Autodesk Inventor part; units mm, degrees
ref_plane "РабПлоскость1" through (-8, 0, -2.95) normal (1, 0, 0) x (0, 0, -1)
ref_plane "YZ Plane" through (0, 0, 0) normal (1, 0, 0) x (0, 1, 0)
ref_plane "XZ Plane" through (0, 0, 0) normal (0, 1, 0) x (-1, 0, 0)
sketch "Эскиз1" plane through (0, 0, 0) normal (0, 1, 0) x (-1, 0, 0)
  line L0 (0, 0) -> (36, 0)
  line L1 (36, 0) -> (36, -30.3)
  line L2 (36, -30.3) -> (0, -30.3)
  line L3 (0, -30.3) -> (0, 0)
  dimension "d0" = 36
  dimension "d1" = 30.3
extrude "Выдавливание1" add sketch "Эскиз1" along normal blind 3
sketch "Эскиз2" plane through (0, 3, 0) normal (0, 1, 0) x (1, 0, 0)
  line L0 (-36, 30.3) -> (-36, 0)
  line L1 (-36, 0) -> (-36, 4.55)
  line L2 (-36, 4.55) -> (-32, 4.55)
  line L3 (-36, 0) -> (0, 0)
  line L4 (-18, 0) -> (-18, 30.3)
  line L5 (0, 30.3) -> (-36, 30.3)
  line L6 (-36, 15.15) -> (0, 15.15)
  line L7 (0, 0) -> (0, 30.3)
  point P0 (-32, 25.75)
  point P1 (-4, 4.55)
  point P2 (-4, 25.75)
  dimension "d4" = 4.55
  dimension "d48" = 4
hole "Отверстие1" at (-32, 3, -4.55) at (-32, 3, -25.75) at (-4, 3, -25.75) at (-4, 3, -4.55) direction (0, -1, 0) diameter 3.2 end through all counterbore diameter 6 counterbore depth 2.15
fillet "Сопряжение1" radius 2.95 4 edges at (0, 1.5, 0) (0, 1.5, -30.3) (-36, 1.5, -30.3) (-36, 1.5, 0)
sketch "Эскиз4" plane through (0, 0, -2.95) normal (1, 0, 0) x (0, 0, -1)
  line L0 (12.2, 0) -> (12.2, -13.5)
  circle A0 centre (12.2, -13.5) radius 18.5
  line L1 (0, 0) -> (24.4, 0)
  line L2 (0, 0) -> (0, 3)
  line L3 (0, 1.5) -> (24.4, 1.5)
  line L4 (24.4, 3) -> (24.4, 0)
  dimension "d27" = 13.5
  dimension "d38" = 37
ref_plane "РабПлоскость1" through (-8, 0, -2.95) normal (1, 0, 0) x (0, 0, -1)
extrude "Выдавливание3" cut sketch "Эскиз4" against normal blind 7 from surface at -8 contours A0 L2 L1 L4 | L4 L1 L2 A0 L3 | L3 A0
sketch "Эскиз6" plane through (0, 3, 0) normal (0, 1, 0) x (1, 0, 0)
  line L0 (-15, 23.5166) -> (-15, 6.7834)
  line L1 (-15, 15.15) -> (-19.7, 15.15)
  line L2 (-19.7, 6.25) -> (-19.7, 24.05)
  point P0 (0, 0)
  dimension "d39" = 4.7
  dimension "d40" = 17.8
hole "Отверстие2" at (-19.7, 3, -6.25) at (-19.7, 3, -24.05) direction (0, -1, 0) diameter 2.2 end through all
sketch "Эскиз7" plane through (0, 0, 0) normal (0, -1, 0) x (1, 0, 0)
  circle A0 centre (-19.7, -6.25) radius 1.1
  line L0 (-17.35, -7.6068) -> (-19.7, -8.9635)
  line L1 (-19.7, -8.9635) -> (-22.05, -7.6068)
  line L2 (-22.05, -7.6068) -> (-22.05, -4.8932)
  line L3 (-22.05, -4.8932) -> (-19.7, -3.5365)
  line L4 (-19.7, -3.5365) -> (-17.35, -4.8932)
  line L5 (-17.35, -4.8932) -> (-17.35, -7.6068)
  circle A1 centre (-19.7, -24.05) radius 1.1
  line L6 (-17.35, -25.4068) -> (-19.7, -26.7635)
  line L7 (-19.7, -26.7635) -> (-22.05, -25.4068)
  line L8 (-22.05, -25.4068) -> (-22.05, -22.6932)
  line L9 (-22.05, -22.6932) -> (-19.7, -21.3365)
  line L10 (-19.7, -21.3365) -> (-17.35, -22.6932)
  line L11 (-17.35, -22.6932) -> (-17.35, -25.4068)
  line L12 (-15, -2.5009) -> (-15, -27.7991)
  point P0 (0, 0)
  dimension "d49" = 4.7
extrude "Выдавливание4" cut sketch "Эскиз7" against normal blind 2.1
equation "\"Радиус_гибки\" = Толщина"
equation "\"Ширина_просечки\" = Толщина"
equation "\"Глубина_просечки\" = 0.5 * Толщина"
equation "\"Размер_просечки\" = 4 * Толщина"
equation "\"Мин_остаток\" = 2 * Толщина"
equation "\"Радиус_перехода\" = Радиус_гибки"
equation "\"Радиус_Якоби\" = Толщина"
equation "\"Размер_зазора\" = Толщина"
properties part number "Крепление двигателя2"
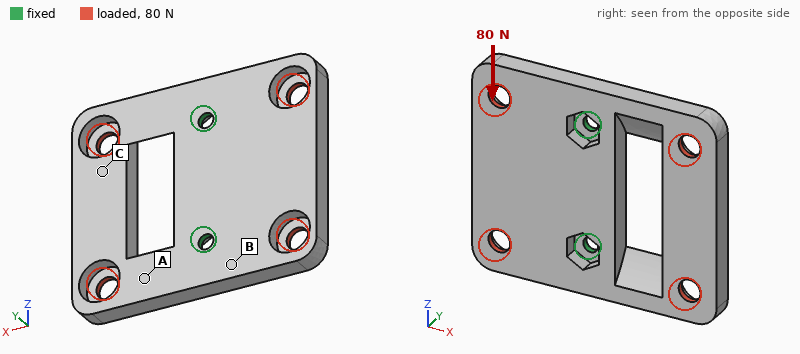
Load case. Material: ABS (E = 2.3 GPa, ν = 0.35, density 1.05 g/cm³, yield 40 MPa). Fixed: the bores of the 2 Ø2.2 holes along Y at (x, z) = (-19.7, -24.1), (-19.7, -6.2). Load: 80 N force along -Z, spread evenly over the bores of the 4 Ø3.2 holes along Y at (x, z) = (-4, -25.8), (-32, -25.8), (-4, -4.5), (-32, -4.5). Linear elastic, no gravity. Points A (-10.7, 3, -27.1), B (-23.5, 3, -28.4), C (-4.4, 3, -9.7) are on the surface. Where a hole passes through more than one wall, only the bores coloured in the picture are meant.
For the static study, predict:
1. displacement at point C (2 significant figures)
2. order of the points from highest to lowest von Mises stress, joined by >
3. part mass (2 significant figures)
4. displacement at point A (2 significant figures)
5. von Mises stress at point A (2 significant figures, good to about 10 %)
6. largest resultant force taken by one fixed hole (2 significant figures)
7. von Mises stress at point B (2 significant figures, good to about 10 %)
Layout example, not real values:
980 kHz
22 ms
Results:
0.11 mm
A > B > C
2.6 g
0.085 mm
4.7 MPa
42 N
2.8 MPa
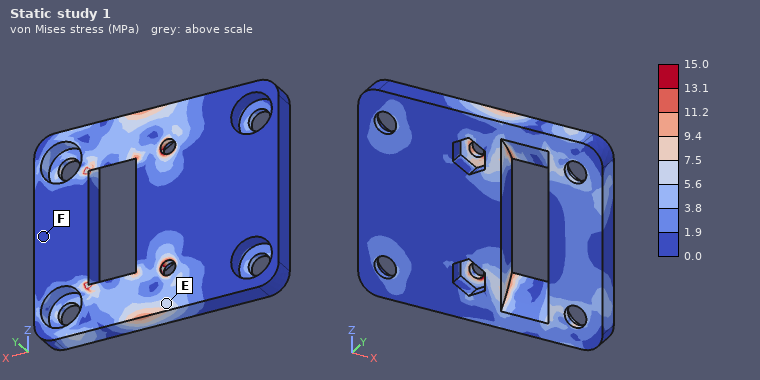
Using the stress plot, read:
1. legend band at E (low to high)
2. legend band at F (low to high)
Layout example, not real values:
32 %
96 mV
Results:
5.6 to 7.5 MPa
0.0 to 1.9 MPa
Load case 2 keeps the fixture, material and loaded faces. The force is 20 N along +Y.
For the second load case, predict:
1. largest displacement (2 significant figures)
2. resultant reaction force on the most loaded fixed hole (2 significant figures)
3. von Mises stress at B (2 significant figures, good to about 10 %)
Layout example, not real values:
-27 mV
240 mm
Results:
0.49 mm
12 N
2.5 MPa
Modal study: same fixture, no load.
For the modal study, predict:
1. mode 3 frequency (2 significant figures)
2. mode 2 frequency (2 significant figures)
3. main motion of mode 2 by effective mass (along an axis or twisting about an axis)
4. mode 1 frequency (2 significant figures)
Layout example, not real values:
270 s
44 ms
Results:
2100 Hz
1700 Hz
along Y
720 Hz
